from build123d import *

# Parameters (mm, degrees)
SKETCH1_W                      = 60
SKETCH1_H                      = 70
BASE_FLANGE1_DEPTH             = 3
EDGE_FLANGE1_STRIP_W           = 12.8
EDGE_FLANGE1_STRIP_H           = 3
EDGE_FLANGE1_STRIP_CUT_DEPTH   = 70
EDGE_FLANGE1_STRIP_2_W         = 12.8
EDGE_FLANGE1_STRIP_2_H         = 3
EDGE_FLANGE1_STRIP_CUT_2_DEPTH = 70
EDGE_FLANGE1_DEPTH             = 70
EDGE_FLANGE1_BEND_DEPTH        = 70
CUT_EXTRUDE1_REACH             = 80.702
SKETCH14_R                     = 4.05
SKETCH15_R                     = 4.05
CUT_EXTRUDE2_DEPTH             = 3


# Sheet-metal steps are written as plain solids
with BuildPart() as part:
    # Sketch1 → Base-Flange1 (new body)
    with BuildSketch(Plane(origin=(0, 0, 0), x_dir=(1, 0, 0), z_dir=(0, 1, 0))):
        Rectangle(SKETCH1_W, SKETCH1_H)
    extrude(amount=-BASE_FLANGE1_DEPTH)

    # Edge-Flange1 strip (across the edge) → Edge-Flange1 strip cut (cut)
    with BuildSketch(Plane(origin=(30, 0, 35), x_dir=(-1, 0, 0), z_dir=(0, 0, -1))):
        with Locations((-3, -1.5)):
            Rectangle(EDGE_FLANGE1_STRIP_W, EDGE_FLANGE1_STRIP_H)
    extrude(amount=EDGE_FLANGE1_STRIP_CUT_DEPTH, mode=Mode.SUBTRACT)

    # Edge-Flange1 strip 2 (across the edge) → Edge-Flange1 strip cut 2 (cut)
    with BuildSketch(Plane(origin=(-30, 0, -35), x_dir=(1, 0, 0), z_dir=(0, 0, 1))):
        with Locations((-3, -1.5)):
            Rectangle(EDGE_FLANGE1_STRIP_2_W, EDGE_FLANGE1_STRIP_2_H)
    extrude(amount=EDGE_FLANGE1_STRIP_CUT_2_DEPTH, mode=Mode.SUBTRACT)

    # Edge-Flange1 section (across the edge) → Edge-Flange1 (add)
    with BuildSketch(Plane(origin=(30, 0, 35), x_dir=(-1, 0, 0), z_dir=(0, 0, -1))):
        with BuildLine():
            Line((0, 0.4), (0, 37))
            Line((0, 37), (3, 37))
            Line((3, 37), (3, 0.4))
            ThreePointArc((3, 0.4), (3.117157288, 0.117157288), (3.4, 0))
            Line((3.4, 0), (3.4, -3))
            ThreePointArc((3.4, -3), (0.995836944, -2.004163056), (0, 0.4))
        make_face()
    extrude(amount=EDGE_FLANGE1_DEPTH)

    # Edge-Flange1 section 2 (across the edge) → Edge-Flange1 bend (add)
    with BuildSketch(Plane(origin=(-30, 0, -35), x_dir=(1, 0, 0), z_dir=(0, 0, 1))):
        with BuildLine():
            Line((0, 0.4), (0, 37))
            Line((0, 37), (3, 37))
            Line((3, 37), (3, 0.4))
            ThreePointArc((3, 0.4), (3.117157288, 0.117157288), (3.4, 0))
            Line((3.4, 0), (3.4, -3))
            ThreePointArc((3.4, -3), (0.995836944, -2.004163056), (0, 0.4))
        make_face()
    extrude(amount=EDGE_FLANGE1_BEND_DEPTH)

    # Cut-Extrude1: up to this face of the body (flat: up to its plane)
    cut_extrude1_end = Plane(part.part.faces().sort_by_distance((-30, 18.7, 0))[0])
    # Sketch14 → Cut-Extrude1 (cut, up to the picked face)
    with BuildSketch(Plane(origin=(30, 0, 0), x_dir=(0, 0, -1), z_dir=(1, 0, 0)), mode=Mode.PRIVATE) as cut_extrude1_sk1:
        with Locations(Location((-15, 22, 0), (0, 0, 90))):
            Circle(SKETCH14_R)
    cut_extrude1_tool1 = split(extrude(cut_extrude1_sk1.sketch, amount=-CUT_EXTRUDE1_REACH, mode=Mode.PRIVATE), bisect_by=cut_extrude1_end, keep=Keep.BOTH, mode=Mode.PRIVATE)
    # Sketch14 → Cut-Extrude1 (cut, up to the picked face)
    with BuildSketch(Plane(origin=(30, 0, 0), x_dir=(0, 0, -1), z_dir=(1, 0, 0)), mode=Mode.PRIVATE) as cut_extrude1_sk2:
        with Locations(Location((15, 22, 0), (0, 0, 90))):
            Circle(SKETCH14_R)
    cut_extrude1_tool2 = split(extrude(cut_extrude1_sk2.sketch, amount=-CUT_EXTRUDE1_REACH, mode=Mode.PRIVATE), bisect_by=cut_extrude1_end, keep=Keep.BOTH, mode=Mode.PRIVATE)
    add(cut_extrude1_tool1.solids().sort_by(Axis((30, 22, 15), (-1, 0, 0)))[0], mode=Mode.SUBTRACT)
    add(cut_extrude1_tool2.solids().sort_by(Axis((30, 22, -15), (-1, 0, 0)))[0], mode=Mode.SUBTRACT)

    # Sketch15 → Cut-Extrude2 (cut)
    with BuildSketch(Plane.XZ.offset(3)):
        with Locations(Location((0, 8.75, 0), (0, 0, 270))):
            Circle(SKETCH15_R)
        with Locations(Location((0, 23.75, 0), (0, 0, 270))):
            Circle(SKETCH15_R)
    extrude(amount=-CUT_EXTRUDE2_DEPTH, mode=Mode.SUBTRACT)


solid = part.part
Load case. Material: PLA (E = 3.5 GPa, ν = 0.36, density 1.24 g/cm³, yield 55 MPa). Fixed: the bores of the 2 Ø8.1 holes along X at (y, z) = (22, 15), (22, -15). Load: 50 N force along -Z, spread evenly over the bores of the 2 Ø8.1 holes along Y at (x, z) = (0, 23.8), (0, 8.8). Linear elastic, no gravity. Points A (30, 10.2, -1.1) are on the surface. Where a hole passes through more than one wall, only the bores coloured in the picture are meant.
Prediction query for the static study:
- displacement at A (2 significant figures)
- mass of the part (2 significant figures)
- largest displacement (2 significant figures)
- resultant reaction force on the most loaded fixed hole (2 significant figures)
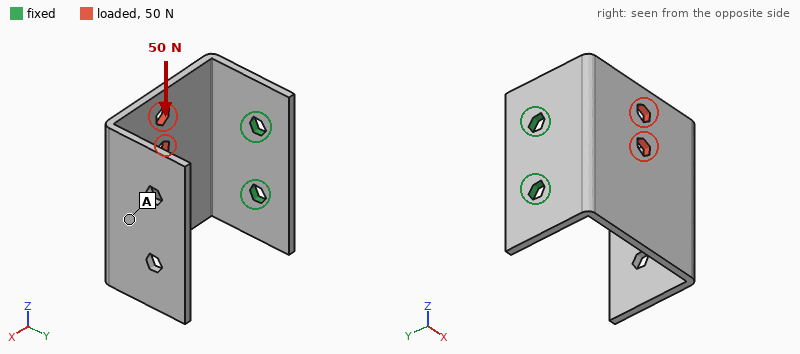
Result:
0.79 mm
33 g
1.1 mm
52 N
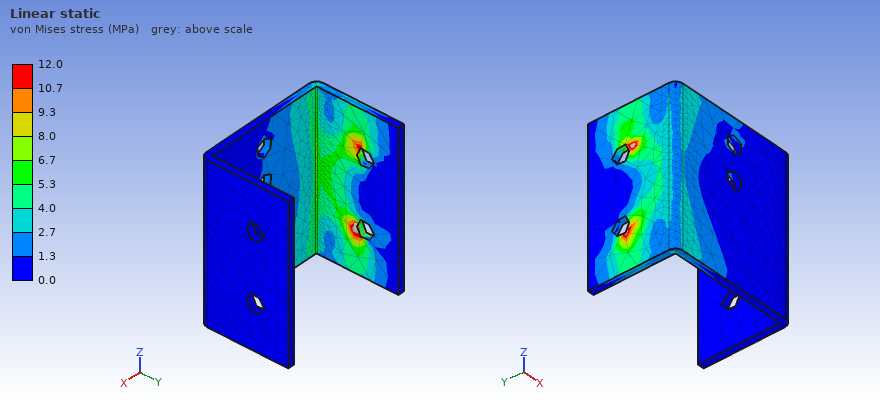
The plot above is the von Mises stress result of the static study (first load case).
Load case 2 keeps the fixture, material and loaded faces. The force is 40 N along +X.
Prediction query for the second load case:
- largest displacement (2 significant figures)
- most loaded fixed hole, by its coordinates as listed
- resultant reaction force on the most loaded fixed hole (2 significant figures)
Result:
1.2 mm
(22, 15)
36 N
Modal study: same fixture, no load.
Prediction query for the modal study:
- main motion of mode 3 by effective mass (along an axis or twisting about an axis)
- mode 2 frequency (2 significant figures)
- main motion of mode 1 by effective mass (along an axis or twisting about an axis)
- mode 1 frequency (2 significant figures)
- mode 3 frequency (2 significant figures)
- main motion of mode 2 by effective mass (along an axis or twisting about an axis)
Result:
along X
160 Hz
along Y
87 Hz
290 Hz
along Z
